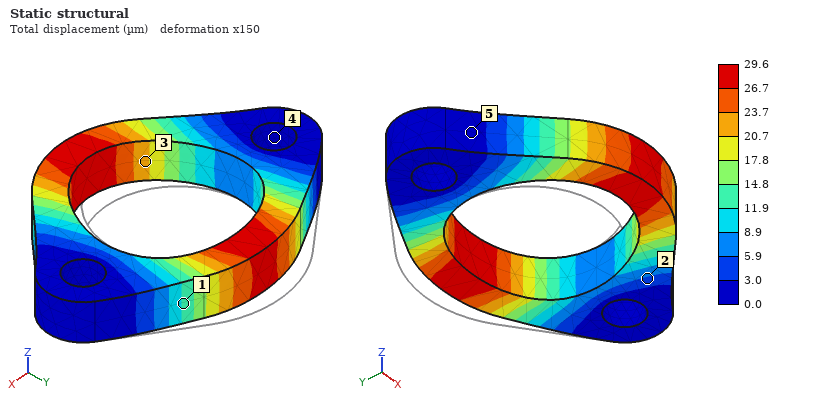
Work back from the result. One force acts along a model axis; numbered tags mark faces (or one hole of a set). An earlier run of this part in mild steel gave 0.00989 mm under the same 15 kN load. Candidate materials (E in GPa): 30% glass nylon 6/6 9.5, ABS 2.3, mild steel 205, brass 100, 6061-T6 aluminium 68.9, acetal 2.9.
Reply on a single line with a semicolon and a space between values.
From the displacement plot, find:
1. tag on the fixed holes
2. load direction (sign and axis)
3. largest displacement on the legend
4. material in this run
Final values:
4; -Y; 29.6 µm; 6061-T6 aluminium
